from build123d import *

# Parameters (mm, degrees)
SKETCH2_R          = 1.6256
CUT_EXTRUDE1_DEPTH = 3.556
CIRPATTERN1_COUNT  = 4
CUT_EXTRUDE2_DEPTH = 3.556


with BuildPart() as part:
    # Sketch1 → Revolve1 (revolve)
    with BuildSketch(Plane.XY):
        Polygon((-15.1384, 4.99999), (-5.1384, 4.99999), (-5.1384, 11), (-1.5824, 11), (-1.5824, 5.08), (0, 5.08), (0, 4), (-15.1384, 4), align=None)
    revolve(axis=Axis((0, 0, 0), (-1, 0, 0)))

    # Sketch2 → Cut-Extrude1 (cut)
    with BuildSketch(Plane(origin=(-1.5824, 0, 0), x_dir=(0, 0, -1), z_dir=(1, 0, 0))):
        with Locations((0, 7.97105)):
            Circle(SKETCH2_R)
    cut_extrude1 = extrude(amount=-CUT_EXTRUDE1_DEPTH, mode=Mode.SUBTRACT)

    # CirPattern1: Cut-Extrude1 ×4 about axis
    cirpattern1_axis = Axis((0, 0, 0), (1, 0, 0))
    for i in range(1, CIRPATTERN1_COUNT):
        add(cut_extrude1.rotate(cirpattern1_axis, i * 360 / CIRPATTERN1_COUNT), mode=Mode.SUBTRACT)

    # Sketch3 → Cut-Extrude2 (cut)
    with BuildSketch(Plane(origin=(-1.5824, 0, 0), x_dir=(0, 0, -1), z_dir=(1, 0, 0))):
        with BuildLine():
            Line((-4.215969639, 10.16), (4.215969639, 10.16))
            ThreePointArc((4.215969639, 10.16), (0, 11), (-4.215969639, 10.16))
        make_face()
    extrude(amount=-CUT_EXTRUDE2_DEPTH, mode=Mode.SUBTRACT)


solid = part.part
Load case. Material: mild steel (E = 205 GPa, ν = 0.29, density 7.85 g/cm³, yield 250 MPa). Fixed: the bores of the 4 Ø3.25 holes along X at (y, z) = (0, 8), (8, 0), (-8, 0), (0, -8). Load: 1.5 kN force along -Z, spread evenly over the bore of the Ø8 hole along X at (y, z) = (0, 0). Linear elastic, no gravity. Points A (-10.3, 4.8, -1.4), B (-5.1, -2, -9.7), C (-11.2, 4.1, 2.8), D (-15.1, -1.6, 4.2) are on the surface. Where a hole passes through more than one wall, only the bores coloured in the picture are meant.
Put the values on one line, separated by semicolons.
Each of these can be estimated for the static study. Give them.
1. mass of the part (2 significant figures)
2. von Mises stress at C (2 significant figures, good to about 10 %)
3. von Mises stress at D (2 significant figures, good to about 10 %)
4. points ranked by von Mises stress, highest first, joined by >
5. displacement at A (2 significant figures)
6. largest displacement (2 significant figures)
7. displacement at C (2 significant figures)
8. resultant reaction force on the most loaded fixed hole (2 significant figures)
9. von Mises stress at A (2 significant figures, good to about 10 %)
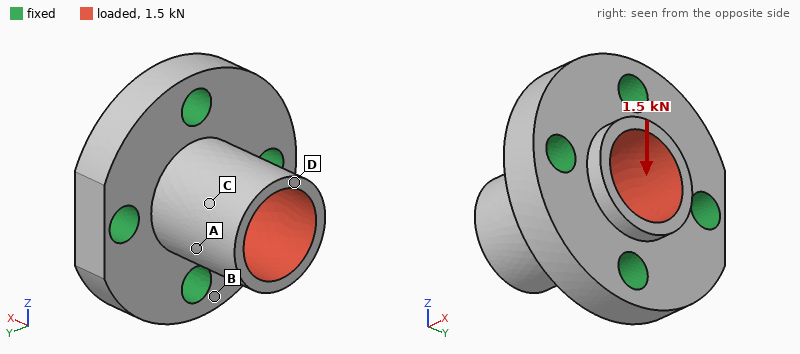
11 g; 39 MPa; 21 MPa; A > C > D > B; 5.6 µm; 9.7 µm; 6.6 µm; 620 N; 53 MPa
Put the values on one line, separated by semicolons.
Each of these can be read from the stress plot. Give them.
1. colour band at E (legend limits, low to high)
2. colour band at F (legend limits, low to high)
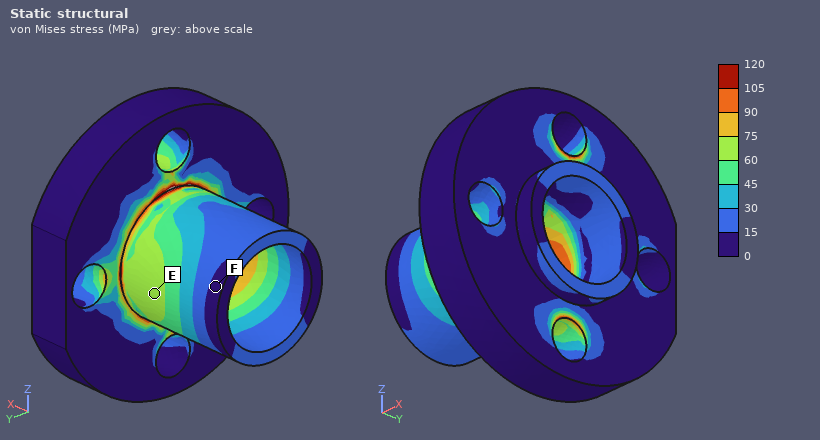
60 to 75 MPa; 0 to 15 MPa
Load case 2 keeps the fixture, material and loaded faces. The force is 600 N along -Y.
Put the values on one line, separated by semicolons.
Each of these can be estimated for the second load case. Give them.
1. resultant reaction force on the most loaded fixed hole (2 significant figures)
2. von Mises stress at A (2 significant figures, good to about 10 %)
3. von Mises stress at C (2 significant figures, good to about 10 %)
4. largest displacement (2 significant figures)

250 N; 11 MPa; 12 MPa; 3.9 µm
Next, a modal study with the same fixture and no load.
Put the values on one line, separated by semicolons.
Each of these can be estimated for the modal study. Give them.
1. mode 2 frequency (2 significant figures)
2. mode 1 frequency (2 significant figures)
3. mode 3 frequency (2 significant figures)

40 kHz; 40 kHz; 40 kHz
